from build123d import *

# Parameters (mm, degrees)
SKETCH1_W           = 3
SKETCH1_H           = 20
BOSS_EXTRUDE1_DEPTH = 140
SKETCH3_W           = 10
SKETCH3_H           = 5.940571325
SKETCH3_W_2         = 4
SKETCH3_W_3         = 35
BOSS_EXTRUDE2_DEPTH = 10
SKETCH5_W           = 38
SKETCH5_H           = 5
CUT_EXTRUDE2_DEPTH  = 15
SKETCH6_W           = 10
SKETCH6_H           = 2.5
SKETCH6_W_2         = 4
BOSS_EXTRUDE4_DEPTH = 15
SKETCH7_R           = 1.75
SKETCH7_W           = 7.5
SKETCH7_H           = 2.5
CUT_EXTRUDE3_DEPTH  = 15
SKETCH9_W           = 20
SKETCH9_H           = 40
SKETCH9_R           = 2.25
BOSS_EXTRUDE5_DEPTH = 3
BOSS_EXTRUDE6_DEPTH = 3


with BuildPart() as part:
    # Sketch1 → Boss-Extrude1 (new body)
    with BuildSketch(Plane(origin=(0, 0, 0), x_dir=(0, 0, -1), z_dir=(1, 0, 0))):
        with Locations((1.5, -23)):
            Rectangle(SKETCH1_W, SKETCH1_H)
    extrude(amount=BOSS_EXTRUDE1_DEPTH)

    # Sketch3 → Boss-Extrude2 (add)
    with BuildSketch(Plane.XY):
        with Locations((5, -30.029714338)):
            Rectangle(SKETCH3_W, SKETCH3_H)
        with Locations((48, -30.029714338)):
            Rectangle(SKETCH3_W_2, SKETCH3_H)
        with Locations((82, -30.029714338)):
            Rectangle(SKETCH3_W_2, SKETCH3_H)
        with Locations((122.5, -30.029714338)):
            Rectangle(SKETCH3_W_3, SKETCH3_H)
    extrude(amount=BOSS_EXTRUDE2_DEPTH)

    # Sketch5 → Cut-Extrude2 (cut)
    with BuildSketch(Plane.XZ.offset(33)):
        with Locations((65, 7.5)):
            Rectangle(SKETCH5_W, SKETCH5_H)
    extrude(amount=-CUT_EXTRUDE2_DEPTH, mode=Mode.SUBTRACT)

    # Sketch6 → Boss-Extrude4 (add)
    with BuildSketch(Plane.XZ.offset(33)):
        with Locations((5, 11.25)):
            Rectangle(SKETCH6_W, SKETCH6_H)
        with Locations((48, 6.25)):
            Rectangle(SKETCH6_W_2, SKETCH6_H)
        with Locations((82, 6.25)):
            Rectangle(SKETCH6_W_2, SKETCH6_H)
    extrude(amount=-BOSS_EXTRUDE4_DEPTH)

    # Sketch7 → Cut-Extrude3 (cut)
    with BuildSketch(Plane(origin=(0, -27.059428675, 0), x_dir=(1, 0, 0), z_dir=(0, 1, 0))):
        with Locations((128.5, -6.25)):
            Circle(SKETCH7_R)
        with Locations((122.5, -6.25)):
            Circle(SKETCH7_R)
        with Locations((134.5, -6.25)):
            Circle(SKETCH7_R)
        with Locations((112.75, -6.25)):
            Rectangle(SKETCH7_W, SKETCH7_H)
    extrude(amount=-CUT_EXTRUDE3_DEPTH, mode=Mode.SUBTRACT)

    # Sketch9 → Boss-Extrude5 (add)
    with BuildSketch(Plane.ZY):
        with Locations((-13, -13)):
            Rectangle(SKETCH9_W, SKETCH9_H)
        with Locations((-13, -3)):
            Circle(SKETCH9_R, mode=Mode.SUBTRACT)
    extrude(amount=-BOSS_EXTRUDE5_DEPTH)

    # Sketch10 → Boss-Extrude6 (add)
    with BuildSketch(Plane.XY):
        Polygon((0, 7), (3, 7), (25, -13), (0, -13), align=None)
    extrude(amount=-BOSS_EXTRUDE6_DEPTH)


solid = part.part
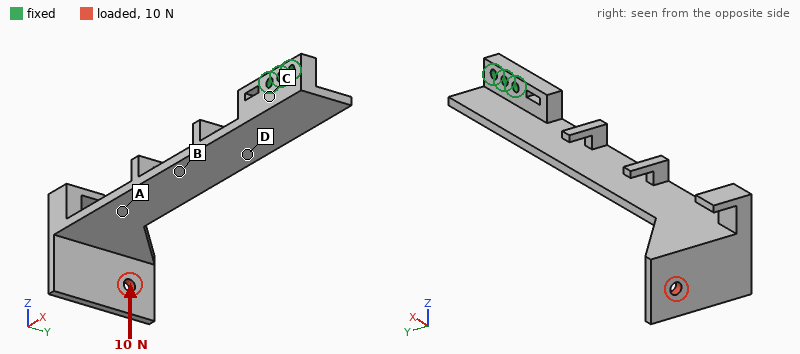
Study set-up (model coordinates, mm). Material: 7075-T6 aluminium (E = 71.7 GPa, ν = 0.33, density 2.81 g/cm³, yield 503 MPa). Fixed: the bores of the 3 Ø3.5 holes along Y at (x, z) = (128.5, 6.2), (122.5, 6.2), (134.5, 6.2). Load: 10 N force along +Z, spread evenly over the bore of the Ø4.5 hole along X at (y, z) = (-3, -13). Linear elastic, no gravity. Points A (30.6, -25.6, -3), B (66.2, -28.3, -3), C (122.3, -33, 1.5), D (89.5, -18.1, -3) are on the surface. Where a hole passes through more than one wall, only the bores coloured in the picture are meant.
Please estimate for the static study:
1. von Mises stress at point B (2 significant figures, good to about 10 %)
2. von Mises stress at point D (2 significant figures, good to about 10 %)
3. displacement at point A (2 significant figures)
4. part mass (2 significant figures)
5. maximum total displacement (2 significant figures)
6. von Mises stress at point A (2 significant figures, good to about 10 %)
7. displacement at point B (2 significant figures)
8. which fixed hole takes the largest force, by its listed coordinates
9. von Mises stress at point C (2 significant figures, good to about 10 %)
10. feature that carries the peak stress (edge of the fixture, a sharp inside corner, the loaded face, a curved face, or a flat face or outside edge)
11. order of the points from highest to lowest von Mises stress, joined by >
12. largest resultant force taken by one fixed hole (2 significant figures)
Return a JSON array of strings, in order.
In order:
["23 MPa", "29 MPa", "0.78 mm", "42 g", "1.5 mm", "11 MPa", "0.27 mm", "(122.5, 6.2)", "5.4 MPa", "a flat face or outside edge", "D > B > A > C", "110 N"]
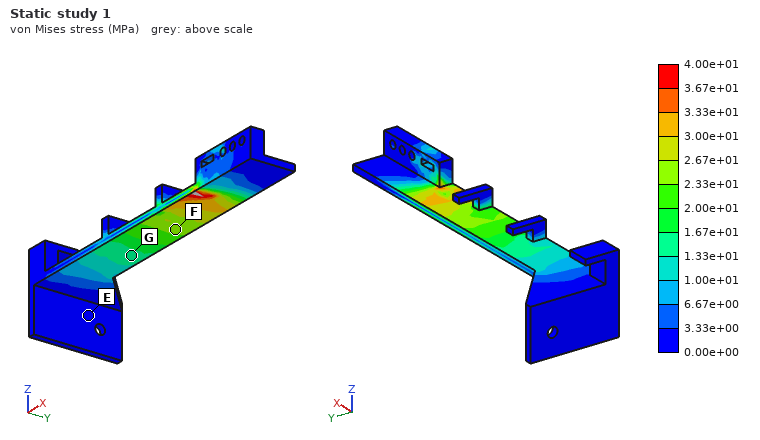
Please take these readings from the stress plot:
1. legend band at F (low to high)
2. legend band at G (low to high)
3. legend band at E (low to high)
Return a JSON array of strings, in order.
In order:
["2.33e+01 to 2.67e+01 MPa", "1.33e+01 to 1.67e+01 MPa", "0.00e+00 to 3.33e+00 MPa"]
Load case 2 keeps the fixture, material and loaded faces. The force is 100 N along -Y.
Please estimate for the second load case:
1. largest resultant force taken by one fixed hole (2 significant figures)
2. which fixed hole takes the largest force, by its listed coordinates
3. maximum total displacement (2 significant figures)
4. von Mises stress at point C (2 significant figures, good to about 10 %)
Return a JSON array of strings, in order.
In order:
["680 N", "(122.5, 6.2)", "1.6 mm", "54 MPa"]
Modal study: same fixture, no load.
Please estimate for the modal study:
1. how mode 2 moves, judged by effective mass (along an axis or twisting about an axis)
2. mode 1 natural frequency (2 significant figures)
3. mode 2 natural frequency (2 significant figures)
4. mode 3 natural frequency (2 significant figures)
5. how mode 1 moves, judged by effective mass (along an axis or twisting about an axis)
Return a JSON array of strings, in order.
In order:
["along Y", "110 Hz", "480 Hz", "620 Hz", "along Z"]
